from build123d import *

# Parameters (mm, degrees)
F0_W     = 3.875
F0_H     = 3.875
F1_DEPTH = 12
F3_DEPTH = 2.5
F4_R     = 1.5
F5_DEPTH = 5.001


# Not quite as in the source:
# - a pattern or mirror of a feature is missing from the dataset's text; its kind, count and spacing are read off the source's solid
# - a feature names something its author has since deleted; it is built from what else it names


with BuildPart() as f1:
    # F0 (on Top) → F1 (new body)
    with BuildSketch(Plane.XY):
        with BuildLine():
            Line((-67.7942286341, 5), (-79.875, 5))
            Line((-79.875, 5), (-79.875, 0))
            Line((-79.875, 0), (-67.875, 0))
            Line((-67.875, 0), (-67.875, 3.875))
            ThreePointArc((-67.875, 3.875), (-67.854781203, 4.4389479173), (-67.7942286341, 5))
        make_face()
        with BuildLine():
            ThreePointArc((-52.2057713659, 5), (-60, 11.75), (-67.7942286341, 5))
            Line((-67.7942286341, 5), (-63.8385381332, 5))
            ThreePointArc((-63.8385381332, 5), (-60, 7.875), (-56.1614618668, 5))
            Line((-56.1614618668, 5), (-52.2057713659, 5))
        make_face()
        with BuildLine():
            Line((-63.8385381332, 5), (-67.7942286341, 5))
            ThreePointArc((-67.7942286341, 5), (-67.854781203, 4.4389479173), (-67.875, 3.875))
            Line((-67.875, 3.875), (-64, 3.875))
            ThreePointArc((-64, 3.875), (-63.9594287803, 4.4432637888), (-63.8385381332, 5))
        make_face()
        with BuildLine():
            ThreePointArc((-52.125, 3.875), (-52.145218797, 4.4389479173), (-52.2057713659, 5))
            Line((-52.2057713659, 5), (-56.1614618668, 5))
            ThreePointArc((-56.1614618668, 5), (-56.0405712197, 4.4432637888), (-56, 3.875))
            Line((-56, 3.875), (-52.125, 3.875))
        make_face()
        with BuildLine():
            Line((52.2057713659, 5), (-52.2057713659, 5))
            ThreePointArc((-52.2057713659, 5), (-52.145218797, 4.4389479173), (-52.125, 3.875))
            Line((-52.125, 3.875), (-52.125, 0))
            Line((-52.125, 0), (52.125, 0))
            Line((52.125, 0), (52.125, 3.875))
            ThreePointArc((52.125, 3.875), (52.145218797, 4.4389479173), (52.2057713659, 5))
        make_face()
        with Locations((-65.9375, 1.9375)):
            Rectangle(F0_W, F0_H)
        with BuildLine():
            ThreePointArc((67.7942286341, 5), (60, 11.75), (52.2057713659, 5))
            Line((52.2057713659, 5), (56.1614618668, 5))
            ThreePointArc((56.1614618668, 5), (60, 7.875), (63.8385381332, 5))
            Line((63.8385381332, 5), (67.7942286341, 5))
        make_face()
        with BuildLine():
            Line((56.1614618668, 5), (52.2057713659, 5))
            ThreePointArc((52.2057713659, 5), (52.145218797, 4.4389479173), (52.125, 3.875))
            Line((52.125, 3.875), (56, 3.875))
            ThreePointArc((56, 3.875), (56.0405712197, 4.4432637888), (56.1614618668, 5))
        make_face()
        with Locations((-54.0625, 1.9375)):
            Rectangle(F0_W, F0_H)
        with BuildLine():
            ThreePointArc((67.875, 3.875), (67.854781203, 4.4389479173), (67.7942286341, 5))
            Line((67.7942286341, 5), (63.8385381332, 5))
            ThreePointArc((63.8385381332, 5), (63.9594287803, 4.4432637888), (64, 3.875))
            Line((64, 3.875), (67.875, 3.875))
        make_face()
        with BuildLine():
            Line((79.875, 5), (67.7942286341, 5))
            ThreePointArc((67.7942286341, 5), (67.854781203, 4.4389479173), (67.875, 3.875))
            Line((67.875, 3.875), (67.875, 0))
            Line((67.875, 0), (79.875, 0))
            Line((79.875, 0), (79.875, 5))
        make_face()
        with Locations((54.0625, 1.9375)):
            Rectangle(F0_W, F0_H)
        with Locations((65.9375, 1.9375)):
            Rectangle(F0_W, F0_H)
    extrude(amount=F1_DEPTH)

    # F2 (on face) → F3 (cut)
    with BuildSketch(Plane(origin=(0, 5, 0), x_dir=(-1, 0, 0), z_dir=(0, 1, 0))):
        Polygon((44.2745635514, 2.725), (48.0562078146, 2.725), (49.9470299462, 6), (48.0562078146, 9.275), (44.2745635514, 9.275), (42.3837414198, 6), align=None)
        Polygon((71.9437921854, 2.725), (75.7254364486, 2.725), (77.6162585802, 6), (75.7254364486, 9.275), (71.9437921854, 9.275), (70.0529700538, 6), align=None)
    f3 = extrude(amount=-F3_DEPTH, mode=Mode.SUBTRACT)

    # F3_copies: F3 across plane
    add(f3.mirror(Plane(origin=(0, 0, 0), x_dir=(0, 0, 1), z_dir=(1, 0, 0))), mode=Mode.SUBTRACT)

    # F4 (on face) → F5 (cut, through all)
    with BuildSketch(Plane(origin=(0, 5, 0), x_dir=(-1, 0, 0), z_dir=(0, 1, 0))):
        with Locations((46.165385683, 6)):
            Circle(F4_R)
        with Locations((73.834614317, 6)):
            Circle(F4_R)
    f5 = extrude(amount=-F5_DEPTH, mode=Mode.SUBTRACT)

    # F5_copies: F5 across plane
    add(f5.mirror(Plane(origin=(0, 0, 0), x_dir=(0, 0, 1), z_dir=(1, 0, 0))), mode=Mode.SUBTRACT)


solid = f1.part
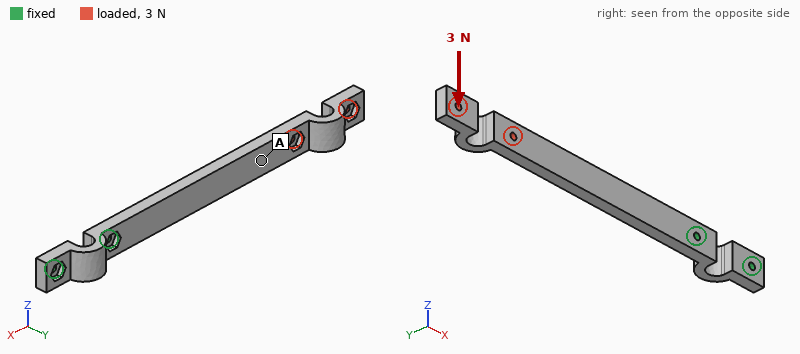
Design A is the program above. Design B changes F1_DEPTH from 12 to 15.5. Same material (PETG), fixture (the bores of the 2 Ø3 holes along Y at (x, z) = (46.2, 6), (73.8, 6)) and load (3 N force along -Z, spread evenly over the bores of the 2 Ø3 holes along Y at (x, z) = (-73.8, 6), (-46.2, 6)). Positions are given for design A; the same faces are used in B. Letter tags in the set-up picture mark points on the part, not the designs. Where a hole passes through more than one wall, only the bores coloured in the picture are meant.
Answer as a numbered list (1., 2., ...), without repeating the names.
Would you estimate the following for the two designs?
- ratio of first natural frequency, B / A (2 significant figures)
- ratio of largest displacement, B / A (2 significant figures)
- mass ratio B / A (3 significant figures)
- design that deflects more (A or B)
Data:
1. 0.99
2. 0.56
3. 1.30
4. A
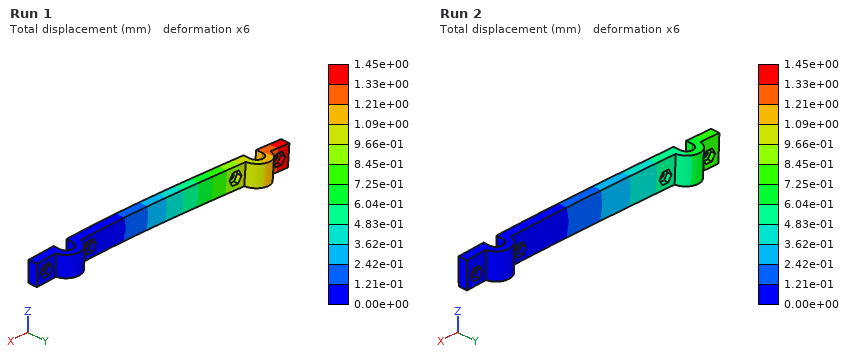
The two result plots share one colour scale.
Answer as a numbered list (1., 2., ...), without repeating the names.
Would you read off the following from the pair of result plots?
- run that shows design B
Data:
1. Run 2
